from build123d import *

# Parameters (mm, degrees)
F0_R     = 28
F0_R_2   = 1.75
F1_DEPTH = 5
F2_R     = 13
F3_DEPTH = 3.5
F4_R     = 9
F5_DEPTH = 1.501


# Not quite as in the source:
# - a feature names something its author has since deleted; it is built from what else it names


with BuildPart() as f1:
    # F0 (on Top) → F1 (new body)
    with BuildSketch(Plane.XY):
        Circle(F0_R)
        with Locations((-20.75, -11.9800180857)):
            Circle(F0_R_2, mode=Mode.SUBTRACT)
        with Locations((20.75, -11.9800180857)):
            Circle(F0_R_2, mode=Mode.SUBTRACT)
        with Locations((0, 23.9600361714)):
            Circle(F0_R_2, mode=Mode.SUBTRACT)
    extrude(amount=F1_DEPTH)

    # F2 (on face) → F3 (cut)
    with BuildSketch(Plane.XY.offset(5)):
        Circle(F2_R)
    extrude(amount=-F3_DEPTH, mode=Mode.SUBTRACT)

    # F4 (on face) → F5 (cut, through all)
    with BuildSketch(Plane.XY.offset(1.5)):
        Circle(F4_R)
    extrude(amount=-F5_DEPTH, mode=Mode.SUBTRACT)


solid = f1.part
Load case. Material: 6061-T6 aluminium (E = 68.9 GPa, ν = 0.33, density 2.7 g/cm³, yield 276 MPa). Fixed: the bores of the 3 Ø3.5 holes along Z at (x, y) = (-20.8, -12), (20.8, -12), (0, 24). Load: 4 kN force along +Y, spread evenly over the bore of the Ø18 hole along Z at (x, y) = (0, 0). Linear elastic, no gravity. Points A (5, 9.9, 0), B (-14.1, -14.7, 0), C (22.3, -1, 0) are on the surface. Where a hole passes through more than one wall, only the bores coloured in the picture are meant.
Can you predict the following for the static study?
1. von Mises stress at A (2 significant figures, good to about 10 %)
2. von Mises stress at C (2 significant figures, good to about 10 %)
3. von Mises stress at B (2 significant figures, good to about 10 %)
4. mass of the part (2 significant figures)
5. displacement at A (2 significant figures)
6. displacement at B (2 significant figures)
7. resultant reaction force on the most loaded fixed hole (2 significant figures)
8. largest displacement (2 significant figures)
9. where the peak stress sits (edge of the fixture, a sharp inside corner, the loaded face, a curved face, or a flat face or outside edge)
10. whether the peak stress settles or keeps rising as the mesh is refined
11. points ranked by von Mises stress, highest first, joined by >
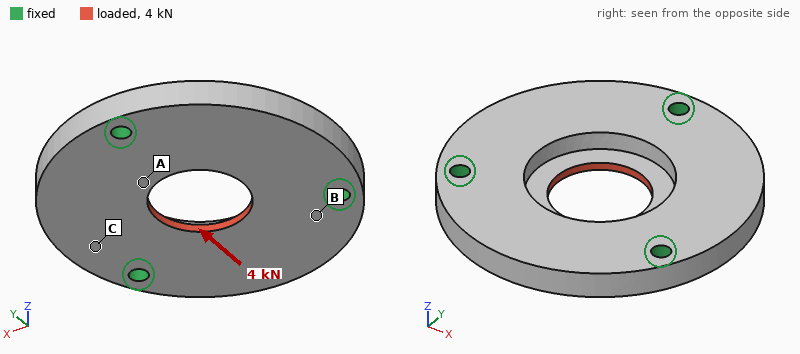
55 MPa
12 MPa
28 MPa
27 g
10 µm
5.6 µm
1.4 kN
19 µm
edge of the fixture
keeps rising
A > B > C
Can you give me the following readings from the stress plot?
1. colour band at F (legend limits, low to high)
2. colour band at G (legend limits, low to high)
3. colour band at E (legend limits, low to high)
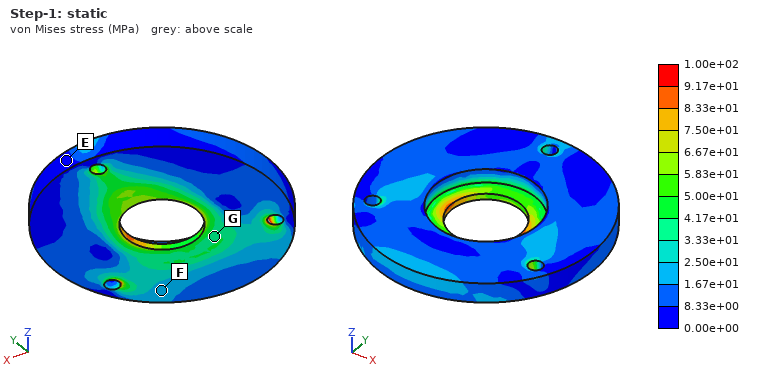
1.67e+01 to 2.50e+01 MPa
3.33e+01 to 4.17e+01 MPa
0.00e+00 to 8.33e+00 MPa
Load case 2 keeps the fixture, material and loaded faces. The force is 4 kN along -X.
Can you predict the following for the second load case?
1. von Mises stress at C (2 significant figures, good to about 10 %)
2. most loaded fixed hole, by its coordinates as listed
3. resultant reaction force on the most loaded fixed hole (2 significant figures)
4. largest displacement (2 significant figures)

19 MPa
(0, 24)
1.5 kN
17 µm
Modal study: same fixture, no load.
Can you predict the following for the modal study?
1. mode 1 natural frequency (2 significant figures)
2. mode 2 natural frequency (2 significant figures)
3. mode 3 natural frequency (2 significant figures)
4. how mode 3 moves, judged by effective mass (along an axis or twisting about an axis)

9500 Hz
9500 Hz
11 kHz
along Z
